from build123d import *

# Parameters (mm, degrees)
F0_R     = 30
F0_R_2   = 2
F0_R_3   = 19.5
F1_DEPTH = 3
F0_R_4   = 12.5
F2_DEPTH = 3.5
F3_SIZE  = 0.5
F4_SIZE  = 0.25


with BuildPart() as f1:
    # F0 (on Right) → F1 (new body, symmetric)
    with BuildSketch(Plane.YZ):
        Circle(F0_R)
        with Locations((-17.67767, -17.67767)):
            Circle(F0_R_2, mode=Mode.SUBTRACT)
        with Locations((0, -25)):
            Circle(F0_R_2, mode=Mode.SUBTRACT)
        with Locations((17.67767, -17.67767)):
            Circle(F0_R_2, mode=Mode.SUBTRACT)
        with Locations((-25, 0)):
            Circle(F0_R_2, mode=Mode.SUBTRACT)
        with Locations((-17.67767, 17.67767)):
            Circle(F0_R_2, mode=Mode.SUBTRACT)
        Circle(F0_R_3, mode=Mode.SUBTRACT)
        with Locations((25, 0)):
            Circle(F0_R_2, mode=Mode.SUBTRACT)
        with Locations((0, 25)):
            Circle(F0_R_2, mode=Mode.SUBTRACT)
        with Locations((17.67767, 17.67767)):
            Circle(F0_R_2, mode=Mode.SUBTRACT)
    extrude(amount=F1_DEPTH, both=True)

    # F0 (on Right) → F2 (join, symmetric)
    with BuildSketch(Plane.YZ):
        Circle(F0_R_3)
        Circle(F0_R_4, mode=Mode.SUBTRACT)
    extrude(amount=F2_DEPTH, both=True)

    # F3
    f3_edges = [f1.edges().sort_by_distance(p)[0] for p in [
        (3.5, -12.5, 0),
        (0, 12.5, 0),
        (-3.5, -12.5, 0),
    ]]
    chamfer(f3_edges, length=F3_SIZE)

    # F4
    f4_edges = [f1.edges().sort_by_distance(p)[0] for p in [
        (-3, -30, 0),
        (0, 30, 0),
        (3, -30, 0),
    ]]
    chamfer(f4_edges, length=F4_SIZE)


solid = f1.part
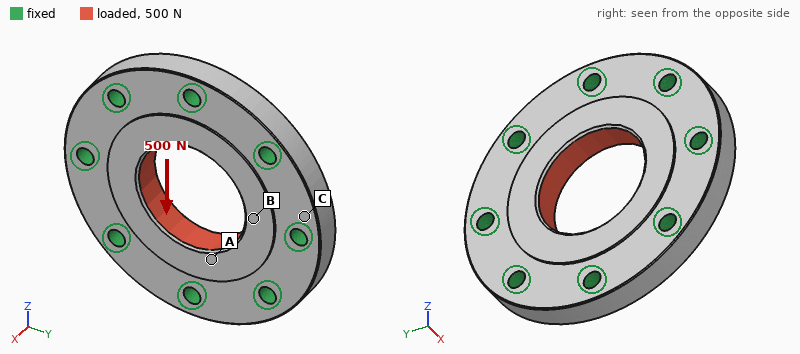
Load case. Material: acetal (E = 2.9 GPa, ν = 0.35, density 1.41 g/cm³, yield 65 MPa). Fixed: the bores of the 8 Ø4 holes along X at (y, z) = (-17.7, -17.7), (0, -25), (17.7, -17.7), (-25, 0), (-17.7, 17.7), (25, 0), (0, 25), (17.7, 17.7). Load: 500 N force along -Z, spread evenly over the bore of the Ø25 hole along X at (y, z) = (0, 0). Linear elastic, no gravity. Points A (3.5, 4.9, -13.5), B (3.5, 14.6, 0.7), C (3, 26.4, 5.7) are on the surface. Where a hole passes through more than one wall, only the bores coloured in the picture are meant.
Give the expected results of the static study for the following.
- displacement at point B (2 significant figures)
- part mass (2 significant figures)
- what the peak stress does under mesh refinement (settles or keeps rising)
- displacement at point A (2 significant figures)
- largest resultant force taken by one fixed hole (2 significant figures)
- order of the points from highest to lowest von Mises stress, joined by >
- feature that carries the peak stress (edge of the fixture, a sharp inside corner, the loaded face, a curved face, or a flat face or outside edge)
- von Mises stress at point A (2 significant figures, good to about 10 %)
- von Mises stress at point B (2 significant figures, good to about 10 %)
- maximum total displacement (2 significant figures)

4.0 µm
20 g
keeps rising
4.5 µm
95 N
B > A > C
edge of the fixture
0.66 MPa
0.88 MPa
5.8 µm
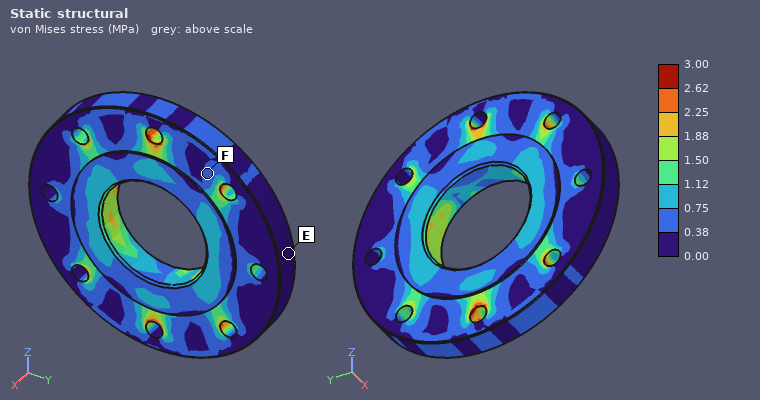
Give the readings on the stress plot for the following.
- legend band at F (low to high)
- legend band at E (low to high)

0.38 to 0.75 MPa
0.00 to 0.38 MPa
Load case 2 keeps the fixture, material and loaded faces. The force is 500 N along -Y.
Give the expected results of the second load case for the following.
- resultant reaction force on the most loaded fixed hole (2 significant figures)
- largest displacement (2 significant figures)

95 N
5.8 µm
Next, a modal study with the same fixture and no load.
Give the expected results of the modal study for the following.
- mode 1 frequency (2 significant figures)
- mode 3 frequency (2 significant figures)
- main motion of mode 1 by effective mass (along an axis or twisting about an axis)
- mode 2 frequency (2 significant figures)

8400 Hz
10 kHz
along X
10 kHz
